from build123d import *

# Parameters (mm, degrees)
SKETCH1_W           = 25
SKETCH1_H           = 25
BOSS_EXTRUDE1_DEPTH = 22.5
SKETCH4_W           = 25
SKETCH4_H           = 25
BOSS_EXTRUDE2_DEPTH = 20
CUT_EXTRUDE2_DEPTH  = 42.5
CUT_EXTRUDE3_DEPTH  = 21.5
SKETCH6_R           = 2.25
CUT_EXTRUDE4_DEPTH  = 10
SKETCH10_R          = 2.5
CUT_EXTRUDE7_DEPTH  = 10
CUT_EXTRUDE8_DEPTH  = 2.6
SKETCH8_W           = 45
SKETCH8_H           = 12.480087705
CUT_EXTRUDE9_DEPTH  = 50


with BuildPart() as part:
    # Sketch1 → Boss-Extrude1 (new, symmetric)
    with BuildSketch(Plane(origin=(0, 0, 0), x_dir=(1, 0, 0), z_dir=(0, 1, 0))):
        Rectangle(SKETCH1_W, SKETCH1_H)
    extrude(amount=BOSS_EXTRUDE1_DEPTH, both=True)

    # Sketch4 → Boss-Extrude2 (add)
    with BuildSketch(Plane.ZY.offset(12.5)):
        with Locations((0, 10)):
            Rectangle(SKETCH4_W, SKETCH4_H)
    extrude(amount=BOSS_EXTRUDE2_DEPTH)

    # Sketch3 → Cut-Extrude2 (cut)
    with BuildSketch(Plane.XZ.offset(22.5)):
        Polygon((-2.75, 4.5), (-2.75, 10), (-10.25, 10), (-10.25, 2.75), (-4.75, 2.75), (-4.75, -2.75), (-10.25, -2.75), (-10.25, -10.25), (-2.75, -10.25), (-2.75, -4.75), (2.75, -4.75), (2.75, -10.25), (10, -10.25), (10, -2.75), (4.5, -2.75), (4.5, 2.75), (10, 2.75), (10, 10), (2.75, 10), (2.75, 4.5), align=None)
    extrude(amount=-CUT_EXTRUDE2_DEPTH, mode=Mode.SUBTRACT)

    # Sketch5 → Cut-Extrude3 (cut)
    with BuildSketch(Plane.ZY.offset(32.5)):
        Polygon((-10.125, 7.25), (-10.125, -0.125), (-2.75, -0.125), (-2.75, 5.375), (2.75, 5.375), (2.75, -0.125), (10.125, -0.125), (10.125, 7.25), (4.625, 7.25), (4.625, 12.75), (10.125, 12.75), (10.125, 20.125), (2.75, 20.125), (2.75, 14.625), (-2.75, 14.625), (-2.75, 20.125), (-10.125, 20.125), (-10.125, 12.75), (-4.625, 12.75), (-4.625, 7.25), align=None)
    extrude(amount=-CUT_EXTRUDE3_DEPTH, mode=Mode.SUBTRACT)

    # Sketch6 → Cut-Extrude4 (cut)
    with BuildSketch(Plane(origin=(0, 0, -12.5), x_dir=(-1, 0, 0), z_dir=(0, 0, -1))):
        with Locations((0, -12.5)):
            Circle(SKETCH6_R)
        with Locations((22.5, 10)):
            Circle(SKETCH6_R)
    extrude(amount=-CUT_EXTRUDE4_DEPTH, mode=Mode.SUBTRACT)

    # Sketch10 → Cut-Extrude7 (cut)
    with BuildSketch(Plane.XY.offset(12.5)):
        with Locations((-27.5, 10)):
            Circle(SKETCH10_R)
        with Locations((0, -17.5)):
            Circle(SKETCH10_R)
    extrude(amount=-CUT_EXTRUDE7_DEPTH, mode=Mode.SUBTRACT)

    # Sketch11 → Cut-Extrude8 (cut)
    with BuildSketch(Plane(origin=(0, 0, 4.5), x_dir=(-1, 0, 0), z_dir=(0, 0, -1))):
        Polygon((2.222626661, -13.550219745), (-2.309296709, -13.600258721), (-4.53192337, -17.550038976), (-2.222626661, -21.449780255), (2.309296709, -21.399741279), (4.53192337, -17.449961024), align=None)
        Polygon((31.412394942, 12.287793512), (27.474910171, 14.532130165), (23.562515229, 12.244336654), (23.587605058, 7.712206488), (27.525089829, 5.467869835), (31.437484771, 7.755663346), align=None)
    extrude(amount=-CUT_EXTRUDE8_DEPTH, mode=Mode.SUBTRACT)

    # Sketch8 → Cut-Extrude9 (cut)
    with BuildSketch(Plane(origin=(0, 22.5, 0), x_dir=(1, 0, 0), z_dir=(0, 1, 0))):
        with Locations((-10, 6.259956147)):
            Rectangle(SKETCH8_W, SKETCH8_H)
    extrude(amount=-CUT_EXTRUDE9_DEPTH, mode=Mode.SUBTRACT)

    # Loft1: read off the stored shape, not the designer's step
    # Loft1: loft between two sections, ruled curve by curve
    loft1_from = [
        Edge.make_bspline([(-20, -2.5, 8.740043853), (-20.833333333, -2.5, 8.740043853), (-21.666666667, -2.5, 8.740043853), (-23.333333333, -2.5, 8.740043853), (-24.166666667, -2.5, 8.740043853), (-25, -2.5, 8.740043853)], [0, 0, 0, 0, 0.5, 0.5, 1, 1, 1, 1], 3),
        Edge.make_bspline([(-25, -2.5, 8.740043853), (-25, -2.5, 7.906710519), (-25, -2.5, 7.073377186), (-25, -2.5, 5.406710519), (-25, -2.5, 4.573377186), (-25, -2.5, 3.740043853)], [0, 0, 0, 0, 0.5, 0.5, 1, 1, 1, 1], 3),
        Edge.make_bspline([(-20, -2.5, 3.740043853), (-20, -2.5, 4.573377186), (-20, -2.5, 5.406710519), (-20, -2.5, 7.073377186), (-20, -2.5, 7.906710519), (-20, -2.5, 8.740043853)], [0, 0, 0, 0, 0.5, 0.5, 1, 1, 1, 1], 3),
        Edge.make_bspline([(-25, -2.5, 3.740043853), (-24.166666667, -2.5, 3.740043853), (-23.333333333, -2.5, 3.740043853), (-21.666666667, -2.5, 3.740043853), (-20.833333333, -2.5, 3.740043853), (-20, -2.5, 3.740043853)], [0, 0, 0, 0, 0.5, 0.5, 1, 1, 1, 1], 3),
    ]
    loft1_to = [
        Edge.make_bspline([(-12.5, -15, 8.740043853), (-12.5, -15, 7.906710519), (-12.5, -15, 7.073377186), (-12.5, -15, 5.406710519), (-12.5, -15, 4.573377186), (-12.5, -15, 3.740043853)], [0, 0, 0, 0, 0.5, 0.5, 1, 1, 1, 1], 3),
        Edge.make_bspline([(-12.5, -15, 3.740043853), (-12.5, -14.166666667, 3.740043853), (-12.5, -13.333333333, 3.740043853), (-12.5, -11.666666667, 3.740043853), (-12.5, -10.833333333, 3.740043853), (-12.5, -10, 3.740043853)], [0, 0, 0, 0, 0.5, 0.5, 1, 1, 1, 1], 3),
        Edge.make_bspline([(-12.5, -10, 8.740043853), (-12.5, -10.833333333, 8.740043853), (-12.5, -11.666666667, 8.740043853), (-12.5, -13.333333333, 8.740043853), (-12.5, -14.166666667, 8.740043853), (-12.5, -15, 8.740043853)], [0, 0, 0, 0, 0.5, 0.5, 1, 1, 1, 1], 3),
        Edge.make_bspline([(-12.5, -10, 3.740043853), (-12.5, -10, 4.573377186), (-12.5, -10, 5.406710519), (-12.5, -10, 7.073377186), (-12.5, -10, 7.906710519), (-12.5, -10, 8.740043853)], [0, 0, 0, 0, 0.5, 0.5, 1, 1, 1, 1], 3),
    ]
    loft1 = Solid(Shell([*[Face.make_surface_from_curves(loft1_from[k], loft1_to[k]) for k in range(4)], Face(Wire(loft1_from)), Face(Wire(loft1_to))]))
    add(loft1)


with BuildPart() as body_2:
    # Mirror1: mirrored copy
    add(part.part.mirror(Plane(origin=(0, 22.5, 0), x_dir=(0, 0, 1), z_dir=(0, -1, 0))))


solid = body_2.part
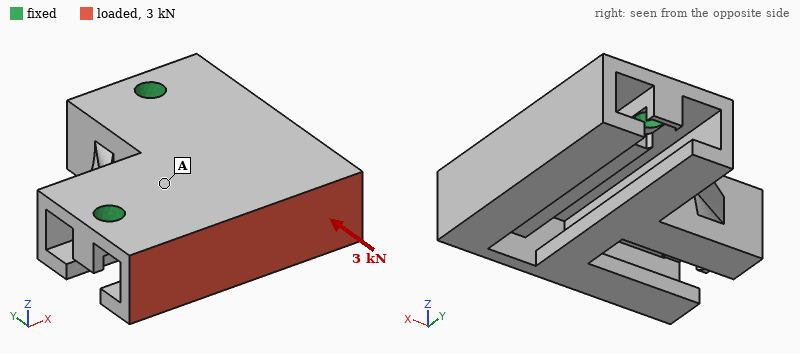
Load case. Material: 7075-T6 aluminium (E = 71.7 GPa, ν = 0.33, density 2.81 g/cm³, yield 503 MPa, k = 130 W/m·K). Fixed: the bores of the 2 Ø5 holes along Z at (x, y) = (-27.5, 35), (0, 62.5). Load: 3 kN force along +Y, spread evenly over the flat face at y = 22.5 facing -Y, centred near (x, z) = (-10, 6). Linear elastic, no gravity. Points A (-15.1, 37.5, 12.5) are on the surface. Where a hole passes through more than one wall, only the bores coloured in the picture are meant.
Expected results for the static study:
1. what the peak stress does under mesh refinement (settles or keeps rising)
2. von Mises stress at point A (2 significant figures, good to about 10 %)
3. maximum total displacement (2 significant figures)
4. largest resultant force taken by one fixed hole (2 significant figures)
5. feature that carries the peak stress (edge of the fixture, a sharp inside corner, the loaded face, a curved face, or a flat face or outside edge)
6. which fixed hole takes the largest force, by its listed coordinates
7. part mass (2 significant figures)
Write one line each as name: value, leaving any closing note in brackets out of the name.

what the peak stress does under mesh refinement: keeps rising
von Mises stress at point A: 20 MPa
maximum total displacement: 0.15 mm
largest resultant force taken by one fixed hole: 1.9 kN
feature that carries the peak stress: edge of the fixture
which fixed hole takes the largest force, by its listed coordinates: (0, 62.5)
part mass: 31 g
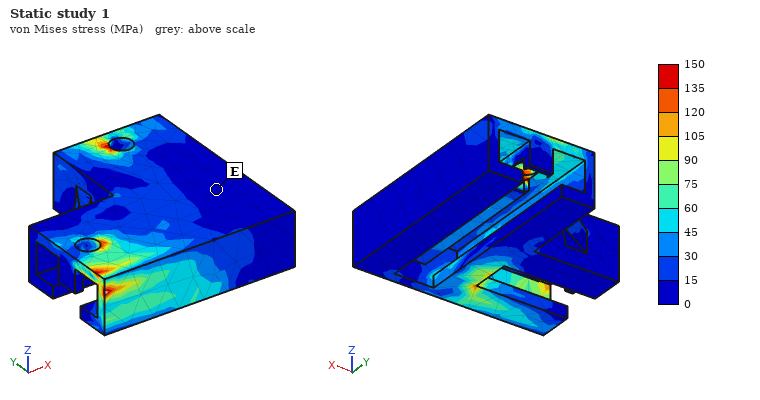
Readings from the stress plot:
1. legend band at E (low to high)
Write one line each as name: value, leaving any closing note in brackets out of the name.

legend band at E: 0 to 15 MPa
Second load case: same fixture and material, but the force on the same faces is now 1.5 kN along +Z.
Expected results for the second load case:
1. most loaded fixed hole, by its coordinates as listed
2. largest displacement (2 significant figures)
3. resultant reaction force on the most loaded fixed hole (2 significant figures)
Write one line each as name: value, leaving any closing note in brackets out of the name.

most loaded fixed hole, by its coordinates as listed: (-27.5, 35)
largest displacement: 0.41 mm
resultant reaction force on the most loaded fixed hole: 1.5 kN
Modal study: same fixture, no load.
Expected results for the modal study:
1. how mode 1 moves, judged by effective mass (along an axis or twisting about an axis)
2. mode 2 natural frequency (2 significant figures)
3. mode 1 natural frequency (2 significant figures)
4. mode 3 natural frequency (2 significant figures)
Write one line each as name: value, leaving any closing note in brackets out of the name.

how mode 1 moves, judged by effective mass: along Z
mode 2 natural frequency: 6500 Hz
mode 1 natural frequency: 3100 Hz
mode 3 natural frequency: 8900 Hz
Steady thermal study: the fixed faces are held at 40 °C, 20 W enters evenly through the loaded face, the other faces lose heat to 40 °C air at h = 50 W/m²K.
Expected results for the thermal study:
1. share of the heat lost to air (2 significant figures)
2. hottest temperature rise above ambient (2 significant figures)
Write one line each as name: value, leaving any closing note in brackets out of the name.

share of the heat lost to air: 17 %
hottest temperature rise above ambient: 20 K
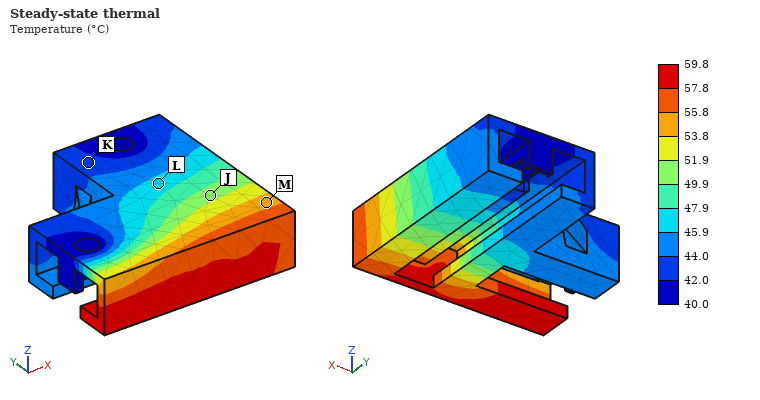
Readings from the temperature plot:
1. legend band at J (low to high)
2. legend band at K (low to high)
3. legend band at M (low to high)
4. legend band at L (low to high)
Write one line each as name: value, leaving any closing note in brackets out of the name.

legend band at J: 49.9 to 51.9 °C
legend band at K: 42.0 to 44.0 °C
legend band at M: 53.8 to 55.8 °C
legend band at L: 45.9 to 47.9 °C
